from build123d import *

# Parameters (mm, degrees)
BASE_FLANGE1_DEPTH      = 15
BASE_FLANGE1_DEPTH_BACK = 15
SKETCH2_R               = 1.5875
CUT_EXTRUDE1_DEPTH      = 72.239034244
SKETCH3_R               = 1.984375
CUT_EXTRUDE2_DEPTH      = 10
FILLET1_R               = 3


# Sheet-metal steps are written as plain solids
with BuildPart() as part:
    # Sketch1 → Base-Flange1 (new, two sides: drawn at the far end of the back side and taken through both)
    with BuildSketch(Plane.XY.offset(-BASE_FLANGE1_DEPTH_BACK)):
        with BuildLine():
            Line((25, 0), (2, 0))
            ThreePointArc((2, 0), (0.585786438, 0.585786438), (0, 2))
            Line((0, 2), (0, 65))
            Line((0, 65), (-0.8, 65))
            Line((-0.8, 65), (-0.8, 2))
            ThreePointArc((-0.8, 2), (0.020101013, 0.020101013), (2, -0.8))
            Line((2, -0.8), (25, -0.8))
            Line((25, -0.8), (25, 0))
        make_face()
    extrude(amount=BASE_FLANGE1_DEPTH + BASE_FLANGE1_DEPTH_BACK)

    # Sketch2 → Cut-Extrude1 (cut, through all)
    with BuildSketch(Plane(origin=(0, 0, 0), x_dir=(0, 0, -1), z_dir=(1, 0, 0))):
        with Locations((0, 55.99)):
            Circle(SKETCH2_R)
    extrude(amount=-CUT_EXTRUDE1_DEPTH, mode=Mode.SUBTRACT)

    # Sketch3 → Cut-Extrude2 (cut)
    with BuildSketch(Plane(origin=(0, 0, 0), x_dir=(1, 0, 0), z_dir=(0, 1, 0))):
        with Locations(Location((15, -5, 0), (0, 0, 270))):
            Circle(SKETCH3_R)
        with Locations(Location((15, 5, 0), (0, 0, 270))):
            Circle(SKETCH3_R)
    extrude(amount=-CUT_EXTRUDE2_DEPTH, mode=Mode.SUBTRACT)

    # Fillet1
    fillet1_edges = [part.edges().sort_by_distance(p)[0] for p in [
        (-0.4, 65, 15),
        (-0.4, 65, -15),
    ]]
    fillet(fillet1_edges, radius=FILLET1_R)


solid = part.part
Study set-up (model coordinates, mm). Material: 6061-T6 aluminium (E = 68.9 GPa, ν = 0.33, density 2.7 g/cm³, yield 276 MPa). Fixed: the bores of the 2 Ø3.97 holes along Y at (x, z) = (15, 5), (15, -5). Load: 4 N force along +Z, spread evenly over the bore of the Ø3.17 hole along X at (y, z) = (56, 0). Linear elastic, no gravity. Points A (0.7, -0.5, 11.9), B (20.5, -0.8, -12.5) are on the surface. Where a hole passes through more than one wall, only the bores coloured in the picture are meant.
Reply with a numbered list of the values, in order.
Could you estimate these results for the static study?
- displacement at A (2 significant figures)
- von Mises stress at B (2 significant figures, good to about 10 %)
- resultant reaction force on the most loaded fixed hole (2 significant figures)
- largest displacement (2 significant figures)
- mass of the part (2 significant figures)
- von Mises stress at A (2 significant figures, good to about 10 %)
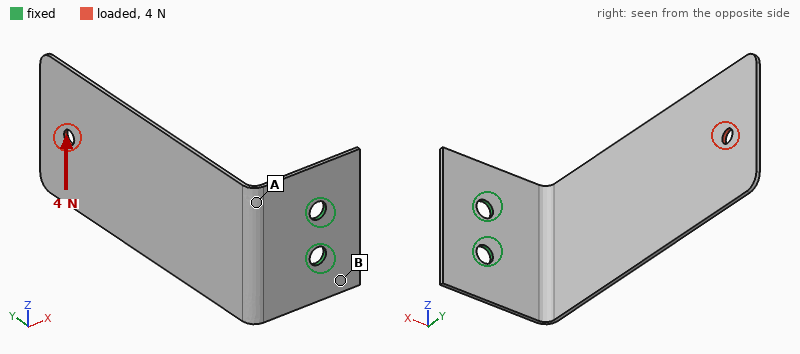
1. 0.13 mm
2. 9.4 MPa
3. 14 N
4. 0.80 mm
5. 5.7 g
6. 29 MPa
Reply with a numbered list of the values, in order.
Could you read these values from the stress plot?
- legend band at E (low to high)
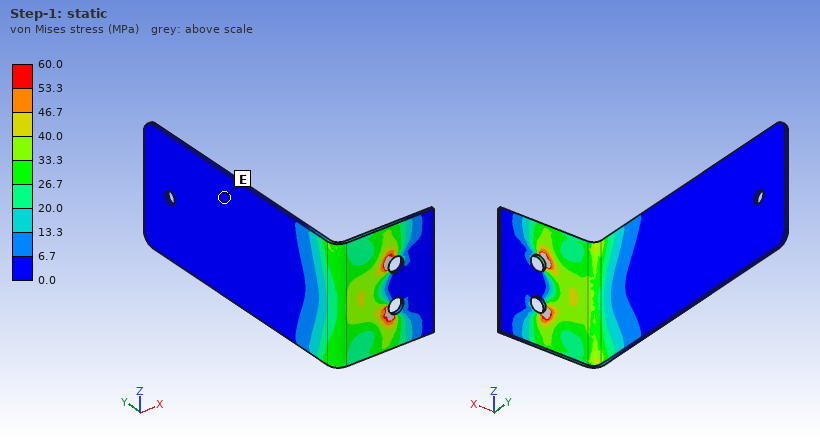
1. 0.0 to 6.7 MPa
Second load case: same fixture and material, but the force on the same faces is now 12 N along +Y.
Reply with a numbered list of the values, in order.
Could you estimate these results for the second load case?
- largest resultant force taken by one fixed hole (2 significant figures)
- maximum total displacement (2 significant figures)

1. 6.0 N
2. 0.88 mm
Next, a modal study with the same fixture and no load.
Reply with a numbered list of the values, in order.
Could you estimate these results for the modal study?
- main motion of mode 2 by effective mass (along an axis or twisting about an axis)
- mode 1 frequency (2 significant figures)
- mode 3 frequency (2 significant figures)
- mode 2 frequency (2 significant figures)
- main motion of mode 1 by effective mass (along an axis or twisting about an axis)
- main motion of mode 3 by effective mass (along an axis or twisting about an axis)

1. along Z
2. 120 Hz
3. 700 Hz
4. 270 Hz
5. along X
6. twisting about Y
